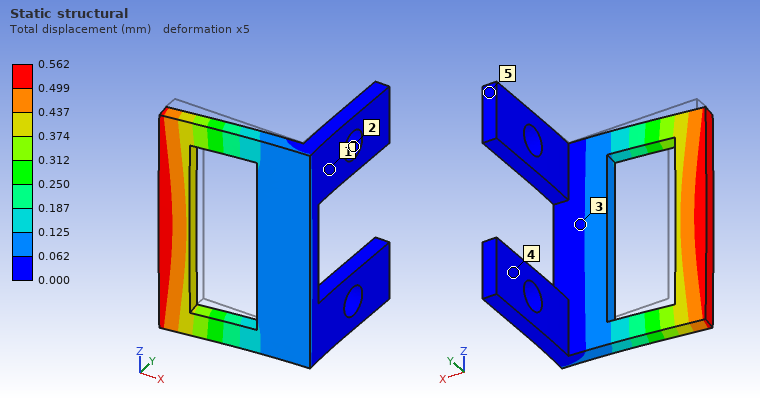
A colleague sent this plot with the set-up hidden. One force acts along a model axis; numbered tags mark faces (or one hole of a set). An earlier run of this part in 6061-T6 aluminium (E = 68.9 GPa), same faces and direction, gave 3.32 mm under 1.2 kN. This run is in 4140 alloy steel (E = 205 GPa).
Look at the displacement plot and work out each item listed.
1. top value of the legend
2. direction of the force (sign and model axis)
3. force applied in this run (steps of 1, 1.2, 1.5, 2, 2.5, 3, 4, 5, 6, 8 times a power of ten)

0.562 mm
-Y
600 N
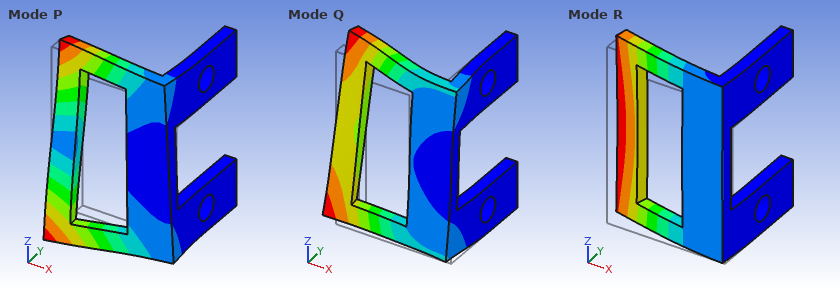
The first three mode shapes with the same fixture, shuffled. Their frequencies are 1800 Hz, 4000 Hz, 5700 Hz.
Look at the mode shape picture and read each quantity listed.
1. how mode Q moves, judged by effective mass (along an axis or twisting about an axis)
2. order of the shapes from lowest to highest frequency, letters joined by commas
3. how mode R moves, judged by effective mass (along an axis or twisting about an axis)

along Z
R, P, Q
along Y
